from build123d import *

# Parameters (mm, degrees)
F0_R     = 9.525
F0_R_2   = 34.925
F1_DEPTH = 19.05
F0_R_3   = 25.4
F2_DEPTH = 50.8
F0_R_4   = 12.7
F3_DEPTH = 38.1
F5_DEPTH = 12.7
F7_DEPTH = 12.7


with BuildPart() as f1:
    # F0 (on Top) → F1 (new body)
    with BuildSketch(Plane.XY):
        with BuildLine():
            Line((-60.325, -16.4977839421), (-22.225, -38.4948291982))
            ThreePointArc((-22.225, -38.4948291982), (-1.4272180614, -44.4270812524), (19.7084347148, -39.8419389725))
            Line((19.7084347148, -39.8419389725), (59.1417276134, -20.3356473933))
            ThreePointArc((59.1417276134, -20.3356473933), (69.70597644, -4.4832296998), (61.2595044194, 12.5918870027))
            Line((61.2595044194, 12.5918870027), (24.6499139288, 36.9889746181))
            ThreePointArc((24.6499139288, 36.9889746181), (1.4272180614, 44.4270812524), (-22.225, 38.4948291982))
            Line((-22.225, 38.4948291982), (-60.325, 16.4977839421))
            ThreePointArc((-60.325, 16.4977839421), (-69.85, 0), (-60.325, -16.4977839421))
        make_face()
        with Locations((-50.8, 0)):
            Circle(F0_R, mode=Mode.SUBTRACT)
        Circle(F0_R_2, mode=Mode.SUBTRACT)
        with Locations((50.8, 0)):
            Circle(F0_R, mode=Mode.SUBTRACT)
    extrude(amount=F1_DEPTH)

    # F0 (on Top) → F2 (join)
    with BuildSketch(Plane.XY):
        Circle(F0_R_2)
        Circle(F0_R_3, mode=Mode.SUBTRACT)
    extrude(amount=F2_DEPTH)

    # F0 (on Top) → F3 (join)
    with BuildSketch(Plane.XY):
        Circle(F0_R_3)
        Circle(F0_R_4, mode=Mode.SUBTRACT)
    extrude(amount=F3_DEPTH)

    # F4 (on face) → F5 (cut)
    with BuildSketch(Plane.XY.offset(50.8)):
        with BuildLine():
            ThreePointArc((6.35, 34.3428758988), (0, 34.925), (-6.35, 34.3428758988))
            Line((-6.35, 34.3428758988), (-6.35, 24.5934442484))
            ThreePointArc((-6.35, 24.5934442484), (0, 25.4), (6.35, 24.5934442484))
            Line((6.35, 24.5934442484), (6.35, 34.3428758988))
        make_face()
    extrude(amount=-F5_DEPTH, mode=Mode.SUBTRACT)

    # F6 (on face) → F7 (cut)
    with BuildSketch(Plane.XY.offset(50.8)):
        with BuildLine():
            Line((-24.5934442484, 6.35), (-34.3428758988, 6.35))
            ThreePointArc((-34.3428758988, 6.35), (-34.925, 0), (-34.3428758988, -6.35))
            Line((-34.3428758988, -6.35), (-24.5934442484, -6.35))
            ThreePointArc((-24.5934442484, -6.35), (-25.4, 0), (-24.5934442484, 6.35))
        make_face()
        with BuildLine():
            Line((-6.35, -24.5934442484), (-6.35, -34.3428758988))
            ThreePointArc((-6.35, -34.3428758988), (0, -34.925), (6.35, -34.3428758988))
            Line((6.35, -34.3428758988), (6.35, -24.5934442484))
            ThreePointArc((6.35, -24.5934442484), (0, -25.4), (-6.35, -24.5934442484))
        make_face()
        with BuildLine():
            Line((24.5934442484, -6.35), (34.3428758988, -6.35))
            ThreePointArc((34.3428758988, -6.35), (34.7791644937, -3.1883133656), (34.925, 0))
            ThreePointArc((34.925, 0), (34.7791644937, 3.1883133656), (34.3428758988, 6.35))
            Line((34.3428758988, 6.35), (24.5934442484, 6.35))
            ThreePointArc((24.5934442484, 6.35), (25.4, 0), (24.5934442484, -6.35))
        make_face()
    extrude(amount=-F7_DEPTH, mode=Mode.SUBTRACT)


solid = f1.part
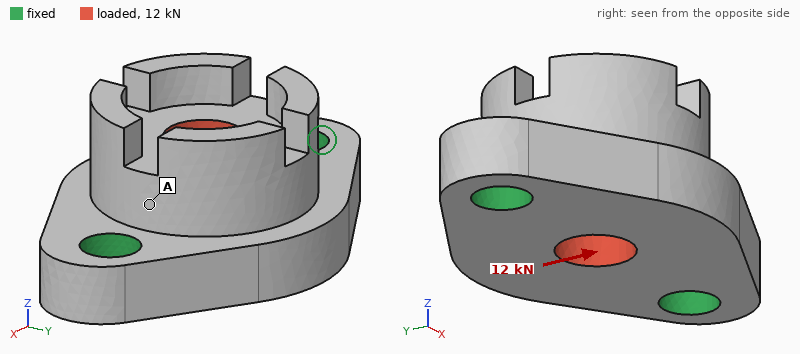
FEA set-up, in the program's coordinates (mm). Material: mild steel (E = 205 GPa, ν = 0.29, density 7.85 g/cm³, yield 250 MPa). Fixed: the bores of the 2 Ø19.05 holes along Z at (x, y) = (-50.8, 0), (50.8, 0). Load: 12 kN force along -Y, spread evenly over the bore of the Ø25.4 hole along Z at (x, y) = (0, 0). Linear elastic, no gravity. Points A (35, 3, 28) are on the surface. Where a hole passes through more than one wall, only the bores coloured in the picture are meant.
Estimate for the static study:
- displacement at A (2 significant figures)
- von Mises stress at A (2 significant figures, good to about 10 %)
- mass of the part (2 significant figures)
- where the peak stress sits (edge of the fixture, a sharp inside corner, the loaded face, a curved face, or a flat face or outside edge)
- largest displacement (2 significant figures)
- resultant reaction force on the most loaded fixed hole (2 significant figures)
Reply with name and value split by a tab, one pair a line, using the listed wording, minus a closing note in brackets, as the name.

displacement at A	3.9 µm
von Mises stress at A	6.3 MPa
mass of the part	1.7 kg
where the peak stress sits	edge of the fixture
largest displacement	8.5 µm
resultant reaction force on the most loaded fixed hole	6.0 kN
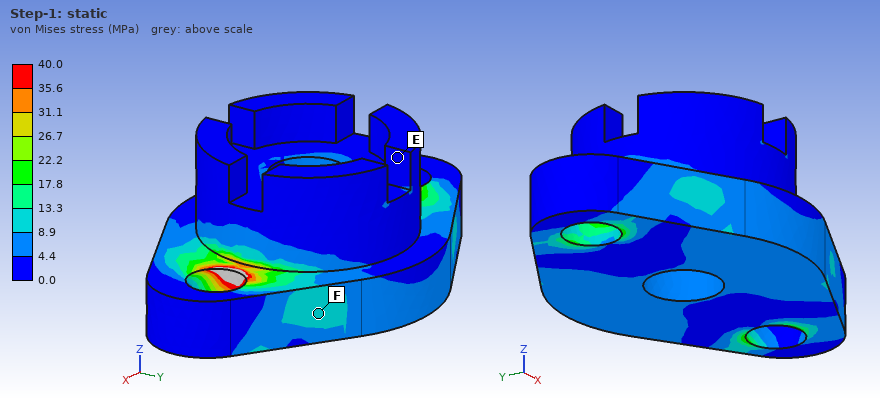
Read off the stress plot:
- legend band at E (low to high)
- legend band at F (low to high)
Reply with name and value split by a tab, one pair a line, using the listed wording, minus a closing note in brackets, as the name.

legend band at E	0.0 to 4.4 MPa
legend band at F	8.9 to 13.3 MPa
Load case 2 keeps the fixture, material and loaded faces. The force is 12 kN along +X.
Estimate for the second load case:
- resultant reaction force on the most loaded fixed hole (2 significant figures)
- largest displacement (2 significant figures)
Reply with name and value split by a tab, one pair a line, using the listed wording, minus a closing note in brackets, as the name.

resultant reaction force on the most loaded fixed hole	6.2 kN
largest displacement	1.8 µm
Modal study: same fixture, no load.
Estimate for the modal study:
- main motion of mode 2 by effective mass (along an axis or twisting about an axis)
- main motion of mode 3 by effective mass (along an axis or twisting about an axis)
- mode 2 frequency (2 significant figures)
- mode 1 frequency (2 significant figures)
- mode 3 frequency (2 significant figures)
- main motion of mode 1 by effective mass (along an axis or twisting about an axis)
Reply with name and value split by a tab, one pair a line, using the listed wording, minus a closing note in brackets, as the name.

main motion of mode 2 by effective mass	along Z
main motion of mode 3 by effective mass	along Y
mode 2 frequency	7300 Hz
mode 1 frequency	4700 Hz
mode 3 frequency	11 kHz
main motion of mode 1 by effective mass	along Y
